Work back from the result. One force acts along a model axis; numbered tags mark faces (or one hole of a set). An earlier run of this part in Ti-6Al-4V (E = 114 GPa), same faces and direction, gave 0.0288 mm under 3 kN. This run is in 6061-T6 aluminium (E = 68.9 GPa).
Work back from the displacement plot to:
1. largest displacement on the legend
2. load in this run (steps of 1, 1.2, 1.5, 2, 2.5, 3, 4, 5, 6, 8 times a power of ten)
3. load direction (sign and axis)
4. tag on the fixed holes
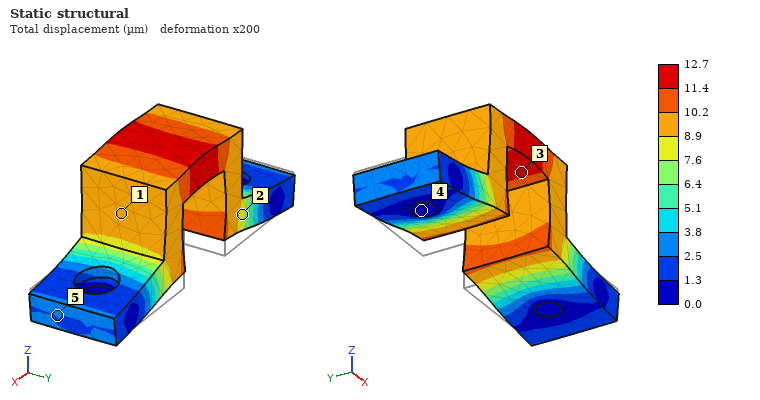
12.7 µm
800 N
+Z
4
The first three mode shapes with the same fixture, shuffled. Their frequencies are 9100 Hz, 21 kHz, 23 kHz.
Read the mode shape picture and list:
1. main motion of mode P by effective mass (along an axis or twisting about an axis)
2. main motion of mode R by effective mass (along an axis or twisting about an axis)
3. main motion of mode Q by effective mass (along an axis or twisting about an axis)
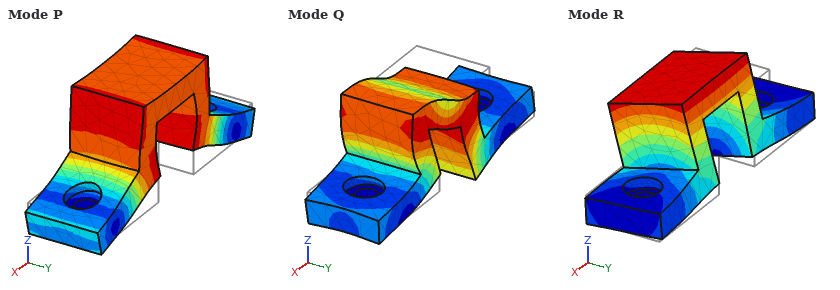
along Z
along Y
along X
